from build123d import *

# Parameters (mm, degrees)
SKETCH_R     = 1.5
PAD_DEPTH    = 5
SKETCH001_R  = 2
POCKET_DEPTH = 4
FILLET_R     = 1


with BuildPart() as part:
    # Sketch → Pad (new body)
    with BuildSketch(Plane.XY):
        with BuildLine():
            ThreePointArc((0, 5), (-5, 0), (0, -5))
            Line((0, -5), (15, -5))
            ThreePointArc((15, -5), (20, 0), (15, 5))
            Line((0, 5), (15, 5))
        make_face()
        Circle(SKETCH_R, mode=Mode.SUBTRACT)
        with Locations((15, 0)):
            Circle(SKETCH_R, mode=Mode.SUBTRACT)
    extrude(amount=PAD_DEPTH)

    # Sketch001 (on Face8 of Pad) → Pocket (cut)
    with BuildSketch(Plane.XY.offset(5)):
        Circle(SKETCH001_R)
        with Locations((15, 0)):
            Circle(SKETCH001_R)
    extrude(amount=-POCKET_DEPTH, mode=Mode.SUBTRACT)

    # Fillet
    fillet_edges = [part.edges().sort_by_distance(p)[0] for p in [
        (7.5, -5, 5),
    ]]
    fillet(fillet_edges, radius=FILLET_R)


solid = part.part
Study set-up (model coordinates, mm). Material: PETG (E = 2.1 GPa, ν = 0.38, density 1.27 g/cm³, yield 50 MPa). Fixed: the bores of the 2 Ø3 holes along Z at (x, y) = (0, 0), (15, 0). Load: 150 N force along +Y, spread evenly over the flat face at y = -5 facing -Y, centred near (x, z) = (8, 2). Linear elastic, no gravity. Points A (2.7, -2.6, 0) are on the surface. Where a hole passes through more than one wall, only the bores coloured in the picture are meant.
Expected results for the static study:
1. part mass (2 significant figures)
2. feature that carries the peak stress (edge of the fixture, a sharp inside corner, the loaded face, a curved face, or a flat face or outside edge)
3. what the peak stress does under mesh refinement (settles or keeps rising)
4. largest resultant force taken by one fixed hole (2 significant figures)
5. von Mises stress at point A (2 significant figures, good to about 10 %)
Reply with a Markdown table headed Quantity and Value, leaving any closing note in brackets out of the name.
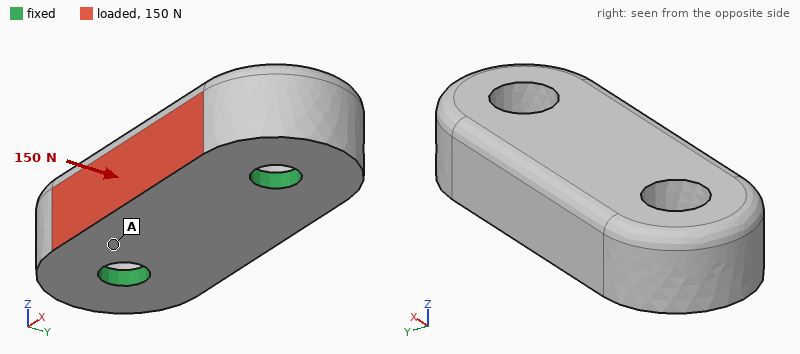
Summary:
| Quantity | Value |
|---|---|
| part mass | 1.3 g |
| feature that carries the peak stress | edge of the fixture |
| what the peak stress does under mesh refinement | keeps rising |
| largest resultant force taken by one fixed hole | 75 N |
| von Mises stress at point A | 6.2 MPa |
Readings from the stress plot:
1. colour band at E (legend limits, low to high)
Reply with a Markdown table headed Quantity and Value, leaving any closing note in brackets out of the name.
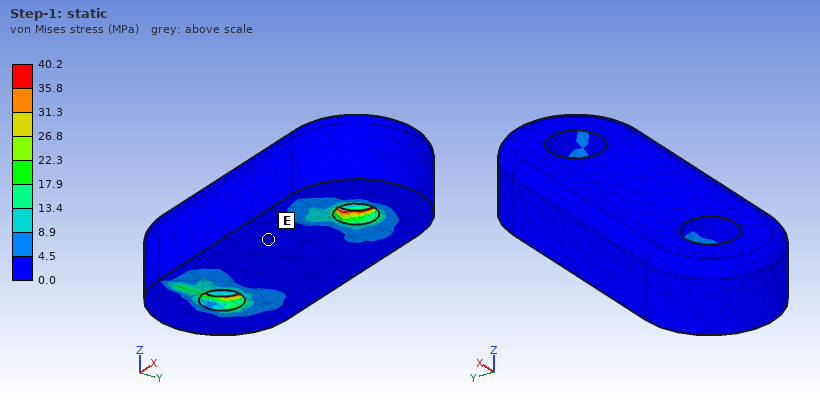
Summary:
| Quantity | Value |
|---|---|
| colour band at E | 0.0 to 4.5 MPa |
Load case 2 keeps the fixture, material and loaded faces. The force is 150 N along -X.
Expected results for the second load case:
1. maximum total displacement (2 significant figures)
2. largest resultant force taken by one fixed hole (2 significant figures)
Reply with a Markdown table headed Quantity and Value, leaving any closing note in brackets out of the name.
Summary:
| Quantity | Value |
|---|---|
| maximum total displacement | 29 µm |
| largest resultant force taken by one fixed hole | 88 N |
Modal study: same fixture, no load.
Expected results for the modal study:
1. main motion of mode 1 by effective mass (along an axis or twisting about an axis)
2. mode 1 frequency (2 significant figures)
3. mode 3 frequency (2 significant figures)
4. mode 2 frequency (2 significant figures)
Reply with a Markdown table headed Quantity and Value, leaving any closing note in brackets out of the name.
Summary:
| Quantity | Value |
|---|---|
| main motion of mode 1 by effective mass | along Y |
| mode 1 frequency | 5500 Hz |
| mode 3 frequency | 12 kHz |
| mode 2 frequency | 12 kHz |
